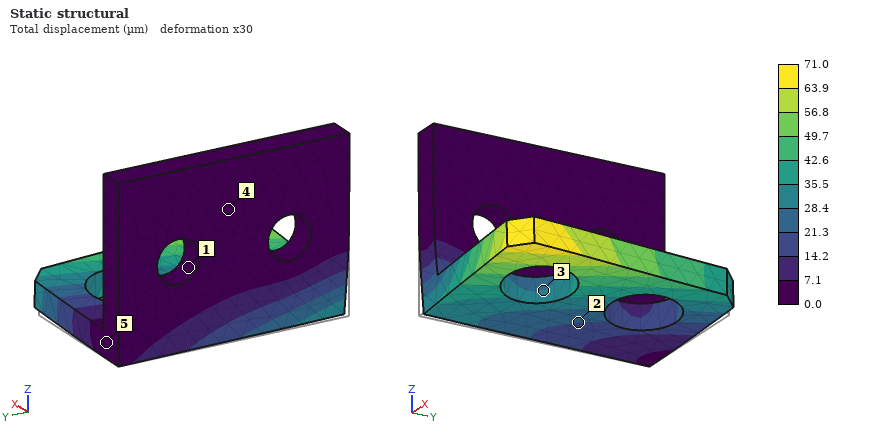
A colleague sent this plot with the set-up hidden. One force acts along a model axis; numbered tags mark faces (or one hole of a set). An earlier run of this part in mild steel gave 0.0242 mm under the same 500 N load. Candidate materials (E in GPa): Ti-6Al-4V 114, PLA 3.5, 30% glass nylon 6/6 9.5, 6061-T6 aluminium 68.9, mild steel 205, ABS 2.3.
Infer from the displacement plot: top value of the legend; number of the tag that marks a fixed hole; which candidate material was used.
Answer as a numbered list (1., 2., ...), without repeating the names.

1. 71.0 µm
2. 1
3. 6061-T6 aluminium
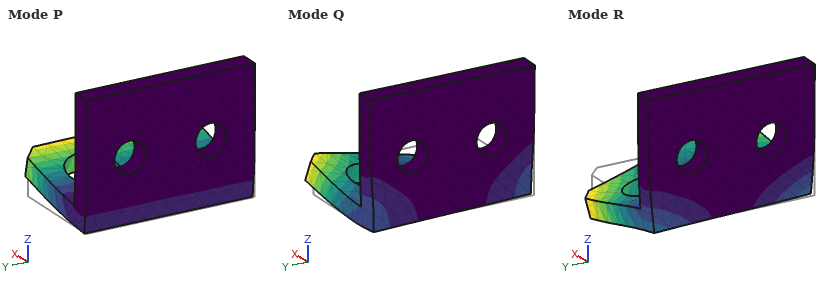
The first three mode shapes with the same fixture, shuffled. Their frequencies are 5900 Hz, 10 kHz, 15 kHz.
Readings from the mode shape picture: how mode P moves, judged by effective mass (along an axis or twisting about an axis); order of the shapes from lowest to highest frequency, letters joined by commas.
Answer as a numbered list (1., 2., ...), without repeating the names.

1. along Z
2. P, R, Q
